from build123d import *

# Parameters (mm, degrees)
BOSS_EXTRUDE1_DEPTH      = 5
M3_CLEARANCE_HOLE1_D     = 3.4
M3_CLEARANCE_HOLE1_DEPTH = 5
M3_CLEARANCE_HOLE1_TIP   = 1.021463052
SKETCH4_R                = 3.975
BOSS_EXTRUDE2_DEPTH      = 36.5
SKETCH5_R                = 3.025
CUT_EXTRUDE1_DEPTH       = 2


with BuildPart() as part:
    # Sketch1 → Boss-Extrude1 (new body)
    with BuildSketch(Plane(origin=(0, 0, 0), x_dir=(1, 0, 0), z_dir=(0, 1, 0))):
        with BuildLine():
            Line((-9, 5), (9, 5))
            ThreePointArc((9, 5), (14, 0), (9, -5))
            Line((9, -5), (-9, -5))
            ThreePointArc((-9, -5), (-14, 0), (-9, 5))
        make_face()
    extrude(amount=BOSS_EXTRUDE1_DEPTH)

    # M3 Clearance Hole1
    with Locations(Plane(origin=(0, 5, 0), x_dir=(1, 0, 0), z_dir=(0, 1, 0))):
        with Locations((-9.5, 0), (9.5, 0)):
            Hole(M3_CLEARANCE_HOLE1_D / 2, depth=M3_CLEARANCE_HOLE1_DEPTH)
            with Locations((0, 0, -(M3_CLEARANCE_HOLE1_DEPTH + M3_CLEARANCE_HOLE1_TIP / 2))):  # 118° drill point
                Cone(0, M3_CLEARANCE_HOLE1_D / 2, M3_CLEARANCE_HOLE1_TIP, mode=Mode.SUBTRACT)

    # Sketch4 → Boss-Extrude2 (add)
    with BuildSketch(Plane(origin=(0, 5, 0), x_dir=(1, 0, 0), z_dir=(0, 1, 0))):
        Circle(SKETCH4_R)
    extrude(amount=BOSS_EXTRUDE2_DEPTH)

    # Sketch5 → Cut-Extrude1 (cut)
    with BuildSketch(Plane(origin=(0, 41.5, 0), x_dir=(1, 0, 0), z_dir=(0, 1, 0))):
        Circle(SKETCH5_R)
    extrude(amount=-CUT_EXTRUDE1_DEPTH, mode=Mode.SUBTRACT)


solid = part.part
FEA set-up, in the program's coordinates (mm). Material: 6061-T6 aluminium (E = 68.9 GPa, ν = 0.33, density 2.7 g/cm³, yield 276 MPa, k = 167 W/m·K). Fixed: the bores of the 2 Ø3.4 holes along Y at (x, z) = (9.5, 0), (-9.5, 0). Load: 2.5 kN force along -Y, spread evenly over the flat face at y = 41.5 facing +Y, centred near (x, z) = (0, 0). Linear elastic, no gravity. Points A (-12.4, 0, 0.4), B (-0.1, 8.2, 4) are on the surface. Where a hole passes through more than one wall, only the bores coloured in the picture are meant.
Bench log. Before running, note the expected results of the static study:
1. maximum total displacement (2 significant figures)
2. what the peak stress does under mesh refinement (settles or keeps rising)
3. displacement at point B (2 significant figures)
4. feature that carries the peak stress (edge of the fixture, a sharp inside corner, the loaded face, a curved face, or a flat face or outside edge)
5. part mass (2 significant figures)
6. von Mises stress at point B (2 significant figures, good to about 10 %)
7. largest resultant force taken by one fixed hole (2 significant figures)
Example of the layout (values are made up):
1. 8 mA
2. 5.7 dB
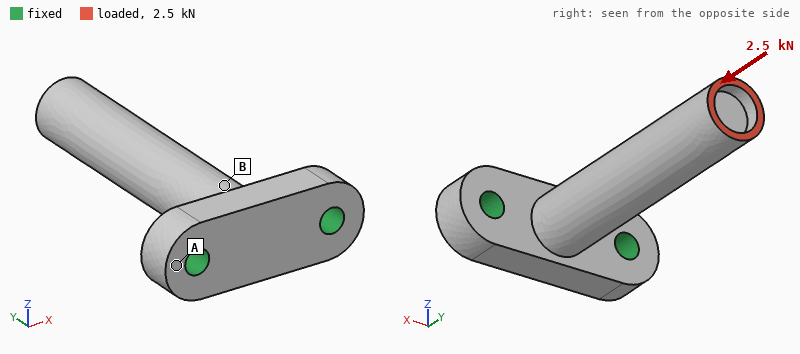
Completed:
1. 44 µm
2. keeps rising
3. 16 µm
4. edge of the fixture
5. 8.0 g
6. 44 MPa
7. 1.3 kN
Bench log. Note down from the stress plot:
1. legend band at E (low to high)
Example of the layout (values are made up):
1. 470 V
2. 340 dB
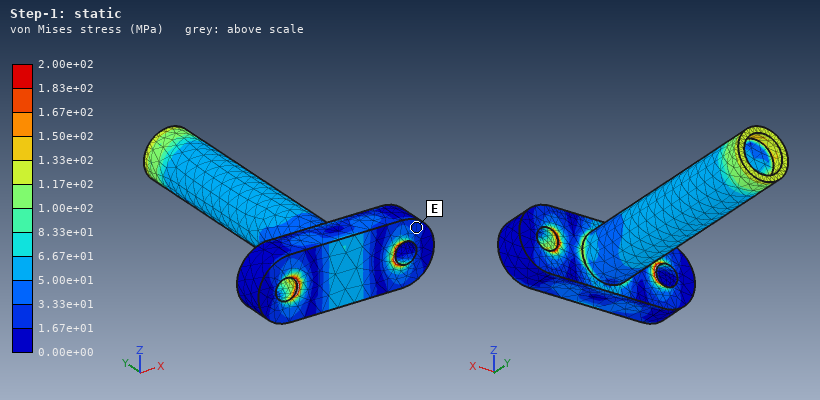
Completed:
1. 1.67e+01 to 3.33e+01 MPa
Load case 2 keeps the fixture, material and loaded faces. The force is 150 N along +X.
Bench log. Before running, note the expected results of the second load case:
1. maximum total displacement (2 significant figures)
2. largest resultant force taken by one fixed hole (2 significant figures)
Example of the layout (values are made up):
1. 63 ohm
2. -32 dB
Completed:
1. 0.23 mm
2. 430 N
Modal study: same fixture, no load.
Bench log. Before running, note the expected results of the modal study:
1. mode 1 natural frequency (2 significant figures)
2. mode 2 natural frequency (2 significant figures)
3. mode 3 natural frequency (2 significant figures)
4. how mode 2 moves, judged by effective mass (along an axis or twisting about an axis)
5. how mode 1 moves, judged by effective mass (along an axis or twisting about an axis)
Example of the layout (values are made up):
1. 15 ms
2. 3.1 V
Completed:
1. 3200 Hz
2. 3800 Hz
3. 19 kHz
4. along X
5. along Z
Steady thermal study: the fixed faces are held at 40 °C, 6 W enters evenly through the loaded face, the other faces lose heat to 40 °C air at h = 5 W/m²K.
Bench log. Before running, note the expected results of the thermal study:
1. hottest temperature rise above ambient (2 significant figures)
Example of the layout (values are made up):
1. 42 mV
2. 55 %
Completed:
1. 32 K
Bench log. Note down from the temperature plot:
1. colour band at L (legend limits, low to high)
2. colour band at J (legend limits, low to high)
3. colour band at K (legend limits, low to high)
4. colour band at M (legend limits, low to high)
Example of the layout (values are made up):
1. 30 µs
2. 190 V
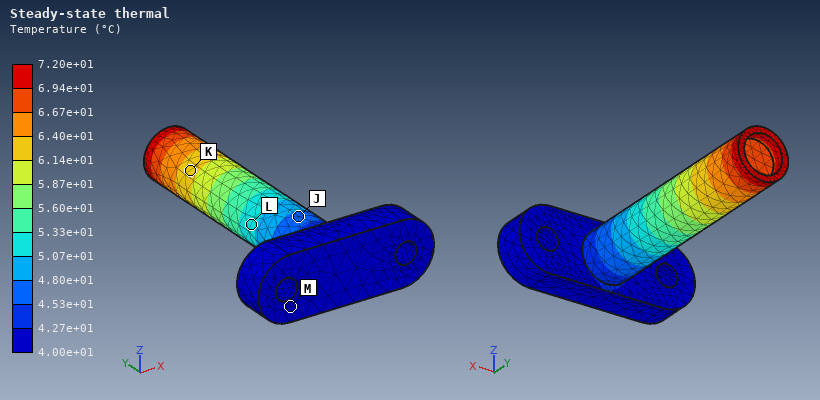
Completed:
1. 5.07e+01 to 5.33e+01 °C
2. 4.53e+01 to 4.80e+01 °C
3. 6.14e+01 to 6.40e+01 °C
4. 4.00e+01 to 4.27e+01 °C
